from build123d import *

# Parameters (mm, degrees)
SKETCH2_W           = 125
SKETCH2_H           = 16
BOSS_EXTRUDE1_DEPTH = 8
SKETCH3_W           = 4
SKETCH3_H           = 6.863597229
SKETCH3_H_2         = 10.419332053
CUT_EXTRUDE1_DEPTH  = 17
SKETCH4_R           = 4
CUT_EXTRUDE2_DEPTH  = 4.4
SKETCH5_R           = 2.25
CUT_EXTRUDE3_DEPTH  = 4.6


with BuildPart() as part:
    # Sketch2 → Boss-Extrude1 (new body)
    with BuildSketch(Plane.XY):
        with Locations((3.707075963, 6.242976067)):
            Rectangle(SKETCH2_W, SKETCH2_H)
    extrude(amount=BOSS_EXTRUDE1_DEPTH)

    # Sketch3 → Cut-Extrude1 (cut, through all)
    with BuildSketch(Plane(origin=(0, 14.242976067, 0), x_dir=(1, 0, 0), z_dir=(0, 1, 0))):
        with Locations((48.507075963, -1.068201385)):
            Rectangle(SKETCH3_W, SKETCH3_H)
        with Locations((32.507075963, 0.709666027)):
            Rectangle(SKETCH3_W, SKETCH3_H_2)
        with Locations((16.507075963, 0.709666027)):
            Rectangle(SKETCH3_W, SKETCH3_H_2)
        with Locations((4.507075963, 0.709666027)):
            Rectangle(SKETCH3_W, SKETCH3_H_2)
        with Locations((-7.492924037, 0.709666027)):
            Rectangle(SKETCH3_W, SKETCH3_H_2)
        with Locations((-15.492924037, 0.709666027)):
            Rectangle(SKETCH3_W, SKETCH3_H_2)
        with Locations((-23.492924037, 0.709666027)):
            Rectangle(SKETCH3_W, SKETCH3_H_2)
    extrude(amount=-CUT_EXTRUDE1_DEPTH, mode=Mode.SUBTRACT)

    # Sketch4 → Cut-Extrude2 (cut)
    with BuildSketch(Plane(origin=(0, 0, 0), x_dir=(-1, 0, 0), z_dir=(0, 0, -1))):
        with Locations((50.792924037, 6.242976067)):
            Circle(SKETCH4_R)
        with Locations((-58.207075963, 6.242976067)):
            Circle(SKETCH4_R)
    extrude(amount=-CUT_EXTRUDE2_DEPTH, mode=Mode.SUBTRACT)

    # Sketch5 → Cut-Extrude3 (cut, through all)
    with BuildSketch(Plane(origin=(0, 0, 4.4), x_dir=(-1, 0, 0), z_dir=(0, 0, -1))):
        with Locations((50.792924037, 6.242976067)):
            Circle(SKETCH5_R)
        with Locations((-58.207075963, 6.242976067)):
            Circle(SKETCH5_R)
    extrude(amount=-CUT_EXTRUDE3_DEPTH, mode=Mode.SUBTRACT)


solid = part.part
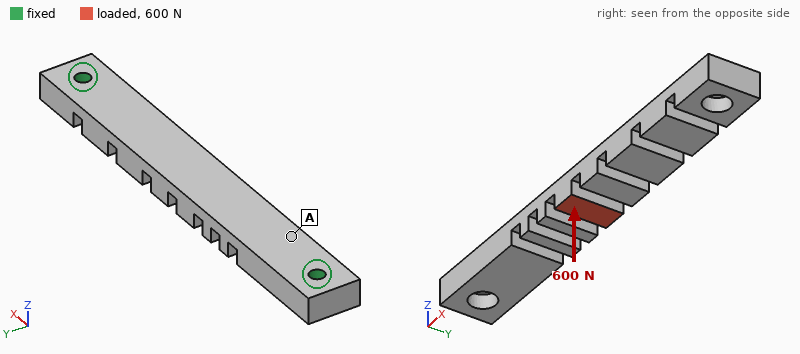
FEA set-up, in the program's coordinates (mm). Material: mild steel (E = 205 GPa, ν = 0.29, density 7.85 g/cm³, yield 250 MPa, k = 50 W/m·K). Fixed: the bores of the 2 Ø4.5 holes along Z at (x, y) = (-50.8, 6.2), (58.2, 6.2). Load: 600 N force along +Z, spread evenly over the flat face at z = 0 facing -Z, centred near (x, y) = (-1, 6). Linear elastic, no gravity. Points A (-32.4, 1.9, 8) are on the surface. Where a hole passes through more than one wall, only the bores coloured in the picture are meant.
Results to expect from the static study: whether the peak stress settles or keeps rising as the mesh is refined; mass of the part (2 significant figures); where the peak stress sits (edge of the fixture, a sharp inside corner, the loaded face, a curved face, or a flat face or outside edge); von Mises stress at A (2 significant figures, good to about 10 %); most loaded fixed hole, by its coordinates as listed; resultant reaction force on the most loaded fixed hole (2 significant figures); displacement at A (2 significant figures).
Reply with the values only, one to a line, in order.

keeps rising
110 g
edge of the fixture
32 MPa
(-50.8, 6.2)
460 N
0.034 mm
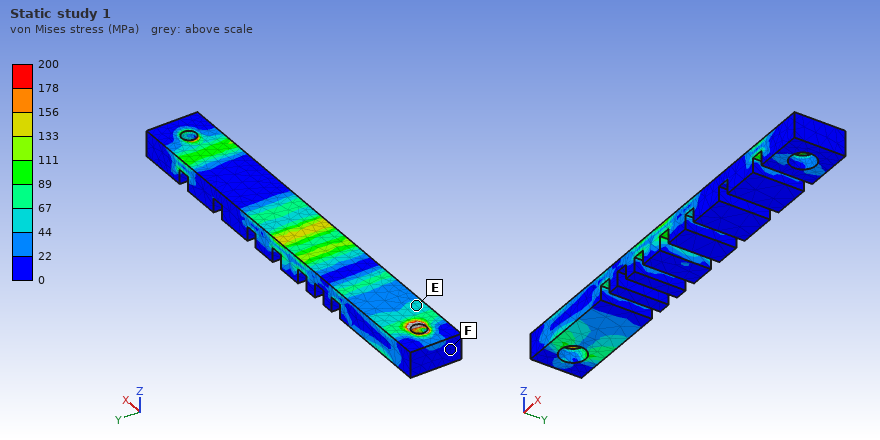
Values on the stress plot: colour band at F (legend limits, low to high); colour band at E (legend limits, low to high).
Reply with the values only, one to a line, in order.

0 to 22 MPa
44 to 67 MPa
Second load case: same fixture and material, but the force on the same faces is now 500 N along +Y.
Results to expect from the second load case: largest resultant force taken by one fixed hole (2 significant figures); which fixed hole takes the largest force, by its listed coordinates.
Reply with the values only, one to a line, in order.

290 N
(-50.8, 6.2)
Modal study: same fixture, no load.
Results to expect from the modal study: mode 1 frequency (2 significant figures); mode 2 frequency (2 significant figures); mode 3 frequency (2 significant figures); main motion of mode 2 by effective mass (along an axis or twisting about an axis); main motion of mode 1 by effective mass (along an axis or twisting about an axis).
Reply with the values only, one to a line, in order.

1800 Hz
4000 Hz
4400 Hz
along Y
along Z
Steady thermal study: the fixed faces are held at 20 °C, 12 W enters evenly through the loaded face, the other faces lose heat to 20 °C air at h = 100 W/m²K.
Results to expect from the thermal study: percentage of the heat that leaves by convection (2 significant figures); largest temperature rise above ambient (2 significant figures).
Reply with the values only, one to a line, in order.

74 %
48 K
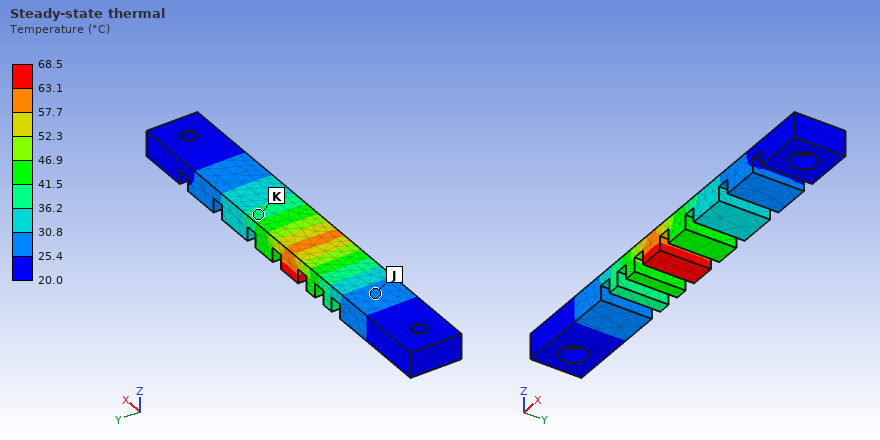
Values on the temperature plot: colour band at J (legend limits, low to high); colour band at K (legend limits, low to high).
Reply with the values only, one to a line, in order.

25.4 to 30.8 °C
36.2 to 41.5 °C
